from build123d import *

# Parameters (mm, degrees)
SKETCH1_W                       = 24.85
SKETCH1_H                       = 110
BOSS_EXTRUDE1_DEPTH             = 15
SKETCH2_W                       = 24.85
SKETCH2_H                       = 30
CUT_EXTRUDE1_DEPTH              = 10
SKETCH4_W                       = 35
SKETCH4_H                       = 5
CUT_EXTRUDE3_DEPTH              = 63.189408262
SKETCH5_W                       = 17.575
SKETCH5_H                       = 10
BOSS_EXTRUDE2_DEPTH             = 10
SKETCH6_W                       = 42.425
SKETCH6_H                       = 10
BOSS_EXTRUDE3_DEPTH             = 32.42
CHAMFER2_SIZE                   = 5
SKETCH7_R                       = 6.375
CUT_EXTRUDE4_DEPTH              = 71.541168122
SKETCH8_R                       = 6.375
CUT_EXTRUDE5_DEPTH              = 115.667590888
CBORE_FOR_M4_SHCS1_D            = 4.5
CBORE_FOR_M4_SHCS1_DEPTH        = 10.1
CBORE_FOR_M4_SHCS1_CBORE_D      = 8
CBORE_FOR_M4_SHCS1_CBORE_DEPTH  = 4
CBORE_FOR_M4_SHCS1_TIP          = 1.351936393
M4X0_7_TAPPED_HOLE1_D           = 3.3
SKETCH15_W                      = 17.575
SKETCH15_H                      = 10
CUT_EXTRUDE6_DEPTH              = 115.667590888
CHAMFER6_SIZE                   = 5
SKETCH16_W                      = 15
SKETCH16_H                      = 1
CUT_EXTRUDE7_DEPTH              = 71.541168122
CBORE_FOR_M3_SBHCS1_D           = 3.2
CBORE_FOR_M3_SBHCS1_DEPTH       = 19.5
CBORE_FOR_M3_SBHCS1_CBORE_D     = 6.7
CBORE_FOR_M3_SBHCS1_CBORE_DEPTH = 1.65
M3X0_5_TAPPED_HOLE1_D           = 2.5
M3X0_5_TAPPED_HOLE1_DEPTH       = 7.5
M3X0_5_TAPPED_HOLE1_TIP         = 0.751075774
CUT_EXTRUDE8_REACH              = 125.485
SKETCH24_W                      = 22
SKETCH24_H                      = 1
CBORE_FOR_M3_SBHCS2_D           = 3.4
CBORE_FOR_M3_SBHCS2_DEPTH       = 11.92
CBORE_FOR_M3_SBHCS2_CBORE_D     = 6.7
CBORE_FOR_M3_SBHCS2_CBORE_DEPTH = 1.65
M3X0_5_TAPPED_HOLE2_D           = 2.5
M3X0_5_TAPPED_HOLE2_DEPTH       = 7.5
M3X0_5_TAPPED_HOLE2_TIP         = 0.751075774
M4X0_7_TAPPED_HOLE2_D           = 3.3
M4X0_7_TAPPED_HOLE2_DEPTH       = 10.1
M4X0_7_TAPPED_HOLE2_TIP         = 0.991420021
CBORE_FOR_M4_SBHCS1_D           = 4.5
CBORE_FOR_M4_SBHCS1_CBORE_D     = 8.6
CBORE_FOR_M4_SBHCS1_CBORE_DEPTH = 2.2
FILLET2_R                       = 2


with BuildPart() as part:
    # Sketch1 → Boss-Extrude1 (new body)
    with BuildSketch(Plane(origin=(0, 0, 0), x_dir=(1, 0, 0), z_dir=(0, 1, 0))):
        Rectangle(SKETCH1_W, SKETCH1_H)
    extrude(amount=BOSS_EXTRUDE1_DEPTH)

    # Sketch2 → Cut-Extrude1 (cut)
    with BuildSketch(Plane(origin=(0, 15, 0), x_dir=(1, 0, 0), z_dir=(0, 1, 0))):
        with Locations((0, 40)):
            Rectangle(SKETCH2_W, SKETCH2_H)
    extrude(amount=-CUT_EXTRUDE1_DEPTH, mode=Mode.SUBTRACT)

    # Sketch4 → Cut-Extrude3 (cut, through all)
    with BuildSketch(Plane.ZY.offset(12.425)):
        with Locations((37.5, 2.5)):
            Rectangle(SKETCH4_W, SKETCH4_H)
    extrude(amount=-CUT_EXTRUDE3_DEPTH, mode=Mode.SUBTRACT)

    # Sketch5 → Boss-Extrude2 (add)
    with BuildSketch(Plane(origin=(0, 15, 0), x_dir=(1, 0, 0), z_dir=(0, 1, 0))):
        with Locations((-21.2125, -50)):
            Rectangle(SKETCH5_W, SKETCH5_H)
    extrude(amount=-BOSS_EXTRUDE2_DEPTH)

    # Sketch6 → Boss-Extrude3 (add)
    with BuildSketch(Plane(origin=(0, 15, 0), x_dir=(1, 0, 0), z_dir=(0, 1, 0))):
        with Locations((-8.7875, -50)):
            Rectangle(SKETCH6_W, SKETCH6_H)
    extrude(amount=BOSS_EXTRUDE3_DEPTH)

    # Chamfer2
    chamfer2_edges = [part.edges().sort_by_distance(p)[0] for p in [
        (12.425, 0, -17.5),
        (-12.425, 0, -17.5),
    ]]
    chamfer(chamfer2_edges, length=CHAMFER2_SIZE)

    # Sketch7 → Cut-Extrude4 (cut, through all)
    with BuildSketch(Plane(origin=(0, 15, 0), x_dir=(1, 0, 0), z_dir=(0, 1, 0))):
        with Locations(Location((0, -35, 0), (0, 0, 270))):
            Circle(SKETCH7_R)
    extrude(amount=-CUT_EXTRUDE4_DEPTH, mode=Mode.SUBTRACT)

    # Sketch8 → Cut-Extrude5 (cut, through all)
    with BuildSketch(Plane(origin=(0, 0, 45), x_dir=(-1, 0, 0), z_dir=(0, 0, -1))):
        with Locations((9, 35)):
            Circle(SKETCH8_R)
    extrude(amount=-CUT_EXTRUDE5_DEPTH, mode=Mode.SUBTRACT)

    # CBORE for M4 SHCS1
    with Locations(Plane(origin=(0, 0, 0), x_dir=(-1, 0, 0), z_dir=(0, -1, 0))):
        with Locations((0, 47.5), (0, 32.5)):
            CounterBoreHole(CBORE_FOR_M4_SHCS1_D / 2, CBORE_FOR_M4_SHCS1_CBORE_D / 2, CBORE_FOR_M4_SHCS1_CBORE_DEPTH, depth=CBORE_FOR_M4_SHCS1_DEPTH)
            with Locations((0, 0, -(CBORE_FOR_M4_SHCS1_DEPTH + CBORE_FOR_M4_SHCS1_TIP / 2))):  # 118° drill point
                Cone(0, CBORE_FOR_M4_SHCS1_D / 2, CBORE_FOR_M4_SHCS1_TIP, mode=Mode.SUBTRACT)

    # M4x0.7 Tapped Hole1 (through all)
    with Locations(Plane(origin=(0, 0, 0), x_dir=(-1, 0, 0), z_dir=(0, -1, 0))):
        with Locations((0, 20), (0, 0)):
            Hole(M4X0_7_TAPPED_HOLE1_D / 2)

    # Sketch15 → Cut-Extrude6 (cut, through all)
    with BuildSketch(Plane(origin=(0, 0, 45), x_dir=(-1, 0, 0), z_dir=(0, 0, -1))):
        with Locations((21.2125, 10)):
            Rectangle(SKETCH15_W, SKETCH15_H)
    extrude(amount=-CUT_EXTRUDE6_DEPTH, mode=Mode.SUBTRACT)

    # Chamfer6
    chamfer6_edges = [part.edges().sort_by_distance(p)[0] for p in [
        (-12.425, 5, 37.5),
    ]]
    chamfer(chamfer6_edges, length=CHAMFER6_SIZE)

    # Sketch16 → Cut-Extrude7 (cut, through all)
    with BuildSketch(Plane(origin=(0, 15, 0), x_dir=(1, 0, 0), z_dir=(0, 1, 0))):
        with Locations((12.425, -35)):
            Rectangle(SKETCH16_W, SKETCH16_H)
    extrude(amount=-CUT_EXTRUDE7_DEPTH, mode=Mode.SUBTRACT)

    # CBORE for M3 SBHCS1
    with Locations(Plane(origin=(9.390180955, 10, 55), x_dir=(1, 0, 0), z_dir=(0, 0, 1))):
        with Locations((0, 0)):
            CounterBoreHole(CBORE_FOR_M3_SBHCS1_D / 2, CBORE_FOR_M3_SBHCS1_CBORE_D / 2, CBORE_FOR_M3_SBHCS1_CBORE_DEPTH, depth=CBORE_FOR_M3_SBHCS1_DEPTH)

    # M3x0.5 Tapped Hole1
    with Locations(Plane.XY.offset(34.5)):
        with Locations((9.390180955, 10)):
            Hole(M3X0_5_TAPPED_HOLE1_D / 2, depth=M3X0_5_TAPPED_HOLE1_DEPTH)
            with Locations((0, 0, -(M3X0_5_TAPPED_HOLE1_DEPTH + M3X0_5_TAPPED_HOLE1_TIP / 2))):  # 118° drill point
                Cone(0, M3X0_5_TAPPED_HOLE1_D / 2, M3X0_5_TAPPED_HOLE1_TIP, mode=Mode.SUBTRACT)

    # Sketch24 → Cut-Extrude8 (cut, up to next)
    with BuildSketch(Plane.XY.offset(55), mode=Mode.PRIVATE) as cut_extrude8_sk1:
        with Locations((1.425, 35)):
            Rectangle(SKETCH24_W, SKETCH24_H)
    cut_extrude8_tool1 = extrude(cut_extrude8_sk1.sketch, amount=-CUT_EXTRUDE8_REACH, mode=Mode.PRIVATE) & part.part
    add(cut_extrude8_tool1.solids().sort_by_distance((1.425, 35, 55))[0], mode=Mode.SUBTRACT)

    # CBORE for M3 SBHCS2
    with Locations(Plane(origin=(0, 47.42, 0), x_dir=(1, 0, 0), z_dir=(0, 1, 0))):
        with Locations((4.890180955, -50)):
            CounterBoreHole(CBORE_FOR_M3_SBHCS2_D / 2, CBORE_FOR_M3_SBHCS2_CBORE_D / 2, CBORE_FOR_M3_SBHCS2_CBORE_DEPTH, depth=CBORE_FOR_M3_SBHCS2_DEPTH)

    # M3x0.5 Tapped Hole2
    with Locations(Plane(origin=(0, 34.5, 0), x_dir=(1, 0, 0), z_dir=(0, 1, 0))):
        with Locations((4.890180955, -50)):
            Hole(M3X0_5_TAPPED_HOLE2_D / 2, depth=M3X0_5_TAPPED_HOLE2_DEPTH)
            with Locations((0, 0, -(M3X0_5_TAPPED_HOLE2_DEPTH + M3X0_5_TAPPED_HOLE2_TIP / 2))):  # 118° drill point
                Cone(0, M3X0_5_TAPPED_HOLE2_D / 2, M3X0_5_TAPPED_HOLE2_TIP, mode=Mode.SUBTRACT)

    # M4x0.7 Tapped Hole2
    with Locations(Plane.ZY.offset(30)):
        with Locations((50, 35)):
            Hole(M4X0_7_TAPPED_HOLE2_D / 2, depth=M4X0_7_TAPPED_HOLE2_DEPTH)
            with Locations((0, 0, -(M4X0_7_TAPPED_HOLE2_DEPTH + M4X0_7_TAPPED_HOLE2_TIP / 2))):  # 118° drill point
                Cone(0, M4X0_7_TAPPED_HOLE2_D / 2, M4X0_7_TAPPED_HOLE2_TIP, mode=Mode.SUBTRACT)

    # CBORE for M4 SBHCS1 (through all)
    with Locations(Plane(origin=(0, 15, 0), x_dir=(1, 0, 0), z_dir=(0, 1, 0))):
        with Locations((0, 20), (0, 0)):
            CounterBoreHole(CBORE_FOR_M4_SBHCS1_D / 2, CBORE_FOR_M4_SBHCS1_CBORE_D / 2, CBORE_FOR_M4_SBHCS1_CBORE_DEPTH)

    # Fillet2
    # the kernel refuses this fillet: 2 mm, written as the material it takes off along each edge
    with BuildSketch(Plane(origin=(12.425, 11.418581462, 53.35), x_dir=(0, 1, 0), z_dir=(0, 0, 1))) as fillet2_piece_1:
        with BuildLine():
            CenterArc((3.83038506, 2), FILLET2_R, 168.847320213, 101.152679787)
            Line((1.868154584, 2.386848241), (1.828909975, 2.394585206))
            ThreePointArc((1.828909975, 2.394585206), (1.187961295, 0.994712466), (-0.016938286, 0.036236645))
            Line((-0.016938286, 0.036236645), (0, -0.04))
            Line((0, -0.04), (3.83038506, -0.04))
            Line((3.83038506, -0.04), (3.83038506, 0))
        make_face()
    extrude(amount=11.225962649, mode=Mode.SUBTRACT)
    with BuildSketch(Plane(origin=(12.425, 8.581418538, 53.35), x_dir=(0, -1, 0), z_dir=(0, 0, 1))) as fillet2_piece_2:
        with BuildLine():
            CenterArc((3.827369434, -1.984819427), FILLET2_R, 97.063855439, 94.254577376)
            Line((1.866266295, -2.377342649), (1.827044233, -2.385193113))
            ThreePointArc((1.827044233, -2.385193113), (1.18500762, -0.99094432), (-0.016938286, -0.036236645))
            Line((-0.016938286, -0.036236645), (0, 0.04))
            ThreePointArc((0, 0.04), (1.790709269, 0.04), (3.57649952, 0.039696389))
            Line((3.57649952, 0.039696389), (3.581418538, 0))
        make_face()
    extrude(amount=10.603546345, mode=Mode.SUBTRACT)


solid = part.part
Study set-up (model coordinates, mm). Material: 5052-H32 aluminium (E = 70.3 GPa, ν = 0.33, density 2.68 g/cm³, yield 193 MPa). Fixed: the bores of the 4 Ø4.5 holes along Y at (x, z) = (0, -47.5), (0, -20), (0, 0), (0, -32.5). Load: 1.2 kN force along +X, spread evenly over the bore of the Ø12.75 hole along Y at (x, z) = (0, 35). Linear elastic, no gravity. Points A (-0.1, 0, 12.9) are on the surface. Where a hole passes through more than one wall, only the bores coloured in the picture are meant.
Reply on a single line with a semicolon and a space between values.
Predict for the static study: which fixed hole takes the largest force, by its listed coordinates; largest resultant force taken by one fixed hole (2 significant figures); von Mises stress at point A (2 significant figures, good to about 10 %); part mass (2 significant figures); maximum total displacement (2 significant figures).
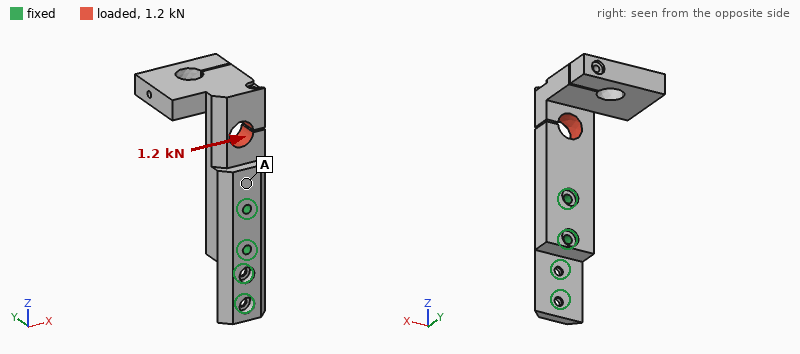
(0, 0); 2.7 kN; 8.5 MPa; 97 g; 0.19 mm
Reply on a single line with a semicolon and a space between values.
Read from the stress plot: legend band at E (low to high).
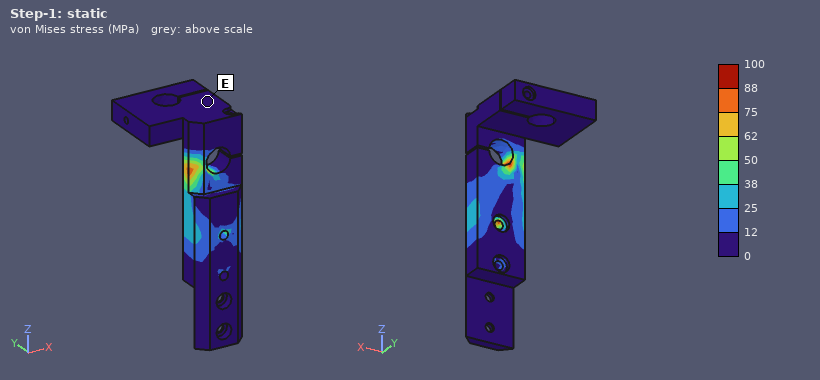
0 to 12 MPa
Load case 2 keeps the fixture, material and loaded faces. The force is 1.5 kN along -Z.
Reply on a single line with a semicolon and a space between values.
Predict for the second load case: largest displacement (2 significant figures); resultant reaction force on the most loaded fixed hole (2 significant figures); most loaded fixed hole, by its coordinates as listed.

0.27 mm; 1.2 kN; (0, 0)
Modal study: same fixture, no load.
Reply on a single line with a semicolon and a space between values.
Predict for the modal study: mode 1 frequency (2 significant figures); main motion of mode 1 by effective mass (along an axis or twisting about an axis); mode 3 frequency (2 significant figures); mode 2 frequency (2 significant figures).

750 Hz; along X; 1400 Hz; 920 Hz
